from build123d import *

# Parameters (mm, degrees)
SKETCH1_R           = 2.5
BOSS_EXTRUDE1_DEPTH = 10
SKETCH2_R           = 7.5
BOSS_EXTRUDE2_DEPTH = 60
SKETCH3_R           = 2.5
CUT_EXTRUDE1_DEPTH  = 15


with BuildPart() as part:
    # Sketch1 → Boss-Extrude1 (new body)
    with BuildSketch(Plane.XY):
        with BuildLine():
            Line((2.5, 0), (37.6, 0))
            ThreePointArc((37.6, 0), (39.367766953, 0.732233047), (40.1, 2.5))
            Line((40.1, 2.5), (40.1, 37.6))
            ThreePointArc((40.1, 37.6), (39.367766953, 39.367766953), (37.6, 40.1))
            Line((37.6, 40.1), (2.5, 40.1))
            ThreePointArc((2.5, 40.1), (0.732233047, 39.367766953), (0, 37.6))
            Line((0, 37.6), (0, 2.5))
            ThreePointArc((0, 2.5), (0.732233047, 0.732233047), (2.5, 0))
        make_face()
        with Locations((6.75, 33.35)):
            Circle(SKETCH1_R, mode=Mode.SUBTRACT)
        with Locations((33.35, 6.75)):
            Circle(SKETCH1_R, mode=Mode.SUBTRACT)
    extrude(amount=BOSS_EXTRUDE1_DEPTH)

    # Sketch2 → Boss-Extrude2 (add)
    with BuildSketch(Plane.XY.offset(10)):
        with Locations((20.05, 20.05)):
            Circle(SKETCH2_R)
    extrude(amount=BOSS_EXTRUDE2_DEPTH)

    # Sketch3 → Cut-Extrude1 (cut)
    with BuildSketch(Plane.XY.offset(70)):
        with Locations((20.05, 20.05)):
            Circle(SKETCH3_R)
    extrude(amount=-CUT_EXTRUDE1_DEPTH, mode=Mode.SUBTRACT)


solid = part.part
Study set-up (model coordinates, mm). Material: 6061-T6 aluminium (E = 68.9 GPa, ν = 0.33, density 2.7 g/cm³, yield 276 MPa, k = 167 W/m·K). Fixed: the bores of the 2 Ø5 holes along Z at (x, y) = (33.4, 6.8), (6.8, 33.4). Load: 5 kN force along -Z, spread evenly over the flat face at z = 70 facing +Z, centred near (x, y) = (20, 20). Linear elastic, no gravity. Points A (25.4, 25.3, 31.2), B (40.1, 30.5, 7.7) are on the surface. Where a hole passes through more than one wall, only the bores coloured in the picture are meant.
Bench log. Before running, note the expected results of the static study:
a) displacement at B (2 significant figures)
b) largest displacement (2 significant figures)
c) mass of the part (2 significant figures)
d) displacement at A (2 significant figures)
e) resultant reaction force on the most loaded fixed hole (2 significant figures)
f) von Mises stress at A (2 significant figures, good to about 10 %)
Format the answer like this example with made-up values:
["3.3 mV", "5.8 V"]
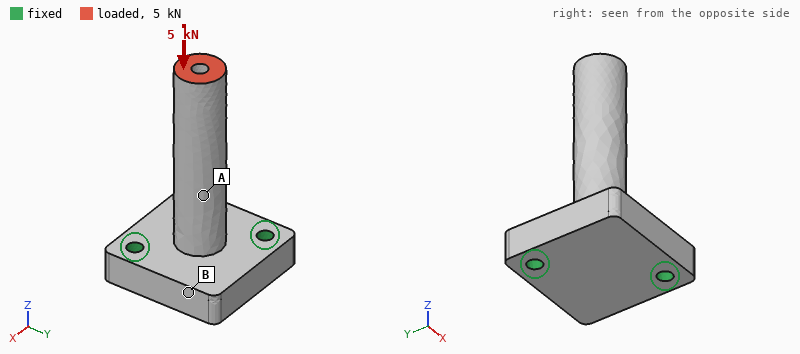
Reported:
["13 µm", "39 µm", "70 g", "22 µm", "2.5 kN", "28 MPa"]
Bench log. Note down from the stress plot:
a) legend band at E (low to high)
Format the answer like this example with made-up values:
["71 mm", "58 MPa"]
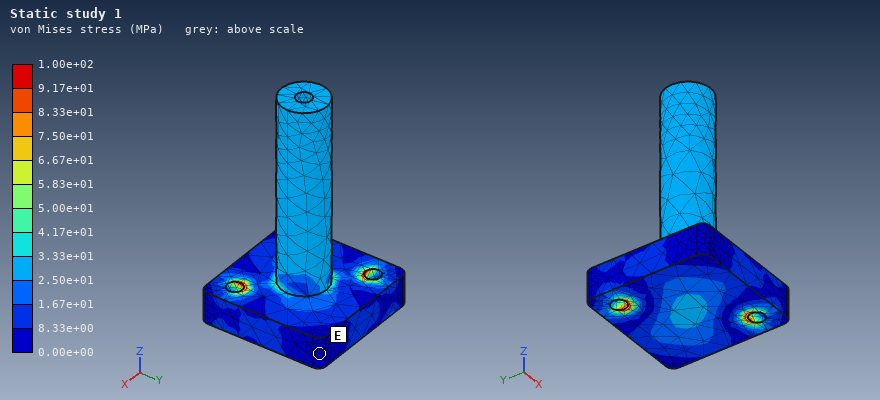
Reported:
["0.00e+00 to 8.33e+00 MPa"]
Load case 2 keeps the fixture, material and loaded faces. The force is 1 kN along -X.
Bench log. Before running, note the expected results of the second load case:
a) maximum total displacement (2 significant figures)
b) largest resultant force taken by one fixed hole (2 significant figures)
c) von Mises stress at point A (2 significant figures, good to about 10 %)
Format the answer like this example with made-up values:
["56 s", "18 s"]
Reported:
["0.61 mm", "1.6 kN", "84 MPa"]
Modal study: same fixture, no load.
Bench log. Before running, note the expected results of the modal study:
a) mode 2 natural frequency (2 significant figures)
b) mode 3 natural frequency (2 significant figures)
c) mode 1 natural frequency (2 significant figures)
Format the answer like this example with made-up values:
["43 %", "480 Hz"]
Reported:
["2600 Hz", "11 kHz", "2300 Hz"]
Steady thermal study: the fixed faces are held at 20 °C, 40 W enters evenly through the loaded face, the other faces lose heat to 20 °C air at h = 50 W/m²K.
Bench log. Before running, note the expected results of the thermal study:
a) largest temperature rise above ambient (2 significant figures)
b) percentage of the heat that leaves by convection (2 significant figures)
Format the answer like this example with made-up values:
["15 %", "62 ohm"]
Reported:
["83 K", "20 %"]
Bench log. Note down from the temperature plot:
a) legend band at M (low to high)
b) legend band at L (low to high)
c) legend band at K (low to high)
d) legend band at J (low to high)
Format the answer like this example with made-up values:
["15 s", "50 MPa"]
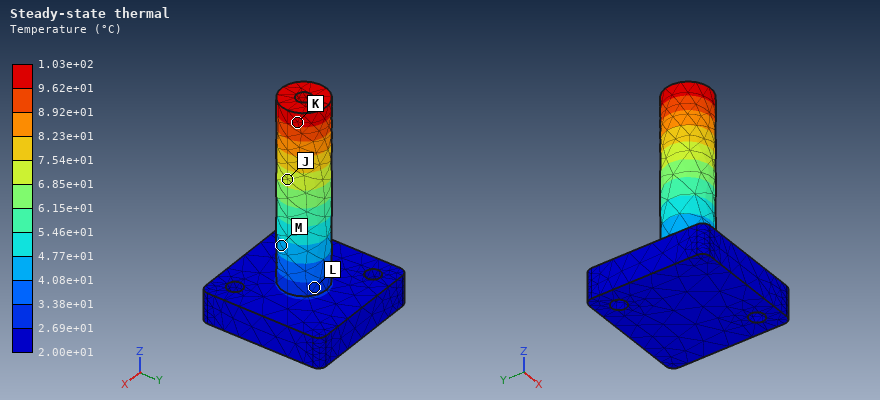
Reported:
["4.08e+01 to 4.77e+01 °C", "2.69e+01 to 3.38e+01 °C", "9.62e+01 to 1.03e+02 °C", "6.85e+01 to 7.54e+01 °C"]
